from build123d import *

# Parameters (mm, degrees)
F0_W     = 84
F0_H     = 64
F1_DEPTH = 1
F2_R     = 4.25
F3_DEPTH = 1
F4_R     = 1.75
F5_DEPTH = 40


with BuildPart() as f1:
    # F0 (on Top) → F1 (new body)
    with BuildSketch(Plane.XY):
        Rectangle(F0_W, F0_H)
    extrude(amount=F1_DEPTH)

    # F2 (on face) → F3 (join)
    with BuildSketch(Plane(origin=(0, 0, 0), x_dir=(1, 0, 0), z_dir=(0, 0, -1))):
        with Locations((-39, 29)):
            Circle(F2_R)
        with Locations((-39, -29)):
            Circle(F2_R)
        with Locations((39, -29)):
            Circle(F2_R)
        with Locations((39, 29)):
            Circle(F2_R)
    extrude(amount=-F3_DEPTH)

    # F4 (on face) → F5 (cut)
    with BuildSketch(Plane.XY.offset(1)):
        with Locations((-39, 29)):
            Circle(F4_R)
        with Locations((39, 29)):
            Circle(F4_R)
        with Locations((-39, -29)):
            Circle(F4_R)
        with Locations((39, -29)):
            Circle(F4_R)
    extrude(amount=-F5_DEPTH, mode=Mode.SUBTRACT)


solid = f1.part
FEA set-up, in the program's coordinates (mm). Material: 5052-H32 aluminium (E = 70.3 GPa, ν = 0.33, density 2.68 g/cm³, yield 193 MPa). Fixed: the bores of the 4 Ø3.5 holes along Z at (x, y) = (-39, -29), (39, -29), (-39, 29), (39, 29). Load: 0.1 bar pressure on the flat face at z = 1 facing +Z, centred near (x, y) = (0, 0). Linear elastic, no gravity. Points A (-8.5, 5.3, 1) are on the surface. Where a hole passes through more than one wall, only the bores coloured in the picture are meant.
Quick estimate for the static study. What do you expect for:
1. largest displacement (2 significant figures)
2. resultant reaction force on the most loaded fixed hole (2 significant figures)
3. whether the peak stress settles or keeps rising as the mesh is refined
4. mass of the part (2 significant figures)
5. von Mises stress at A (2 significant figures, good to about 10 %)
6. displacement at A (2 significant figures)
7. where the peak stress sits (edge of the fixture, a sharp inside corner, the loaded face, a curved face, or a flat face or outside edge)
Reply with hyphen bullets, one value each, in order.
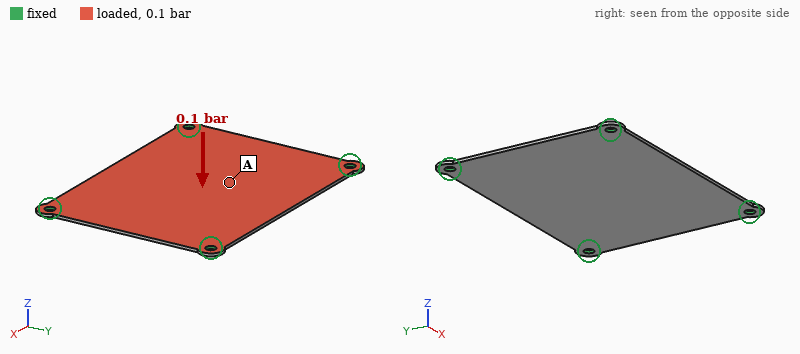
- 0.28 mm
- 13 N
- keeps rising
- 14 g
- 15 MPa
- 0.26 mm
- edge of the fixture
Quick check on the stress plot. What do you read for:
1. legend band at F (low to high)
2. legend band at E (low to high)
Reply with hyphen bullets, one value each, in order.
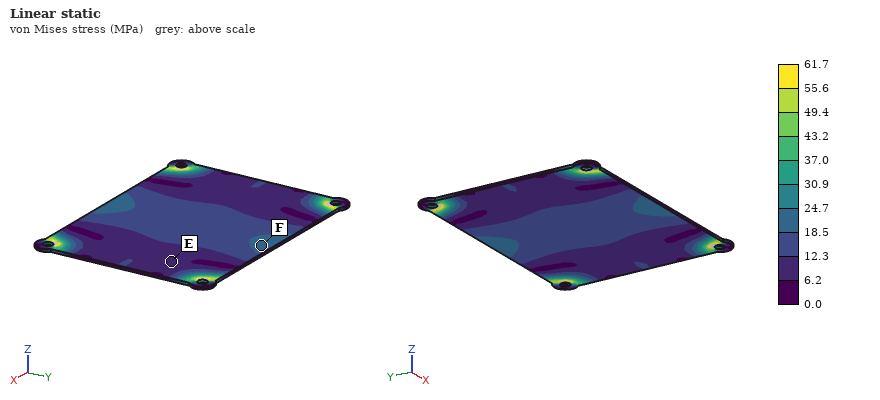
- 18.5 to 24.7 MPa
- 6.2 to 12.3 MPa
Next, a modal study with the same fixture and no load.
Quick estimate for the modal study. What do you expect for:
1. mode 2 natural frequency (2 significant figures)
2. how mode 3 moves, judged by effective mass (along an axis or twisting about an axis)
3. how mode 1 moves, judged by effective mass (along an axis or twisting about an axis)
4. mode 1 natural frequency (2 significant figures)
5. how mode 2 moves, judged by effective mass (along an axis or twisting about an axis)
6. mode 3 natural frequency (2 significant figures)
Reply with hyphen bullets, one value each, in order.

- 1100 Hz
- twisting about Y
- along Z
- 680 Hz
- twisting about X
- 1500 Hz
